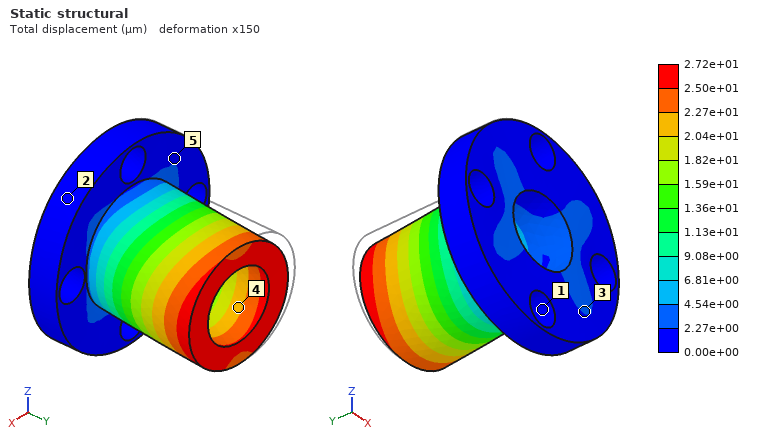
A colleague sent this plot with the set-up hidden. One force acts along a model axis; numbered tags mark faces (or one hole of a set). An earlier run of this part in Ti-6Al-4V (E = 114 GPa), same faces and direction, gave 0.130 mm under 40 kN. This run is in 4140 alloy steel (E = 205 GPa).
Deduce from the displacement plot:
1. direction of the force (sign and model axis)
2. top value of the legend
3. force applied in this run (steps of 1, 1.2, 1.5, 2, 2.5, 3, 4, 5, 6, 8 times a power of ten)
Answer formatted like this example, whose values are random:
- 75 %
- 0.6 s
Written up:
- +X
- 2.72e+01 µm
- 15 kN
